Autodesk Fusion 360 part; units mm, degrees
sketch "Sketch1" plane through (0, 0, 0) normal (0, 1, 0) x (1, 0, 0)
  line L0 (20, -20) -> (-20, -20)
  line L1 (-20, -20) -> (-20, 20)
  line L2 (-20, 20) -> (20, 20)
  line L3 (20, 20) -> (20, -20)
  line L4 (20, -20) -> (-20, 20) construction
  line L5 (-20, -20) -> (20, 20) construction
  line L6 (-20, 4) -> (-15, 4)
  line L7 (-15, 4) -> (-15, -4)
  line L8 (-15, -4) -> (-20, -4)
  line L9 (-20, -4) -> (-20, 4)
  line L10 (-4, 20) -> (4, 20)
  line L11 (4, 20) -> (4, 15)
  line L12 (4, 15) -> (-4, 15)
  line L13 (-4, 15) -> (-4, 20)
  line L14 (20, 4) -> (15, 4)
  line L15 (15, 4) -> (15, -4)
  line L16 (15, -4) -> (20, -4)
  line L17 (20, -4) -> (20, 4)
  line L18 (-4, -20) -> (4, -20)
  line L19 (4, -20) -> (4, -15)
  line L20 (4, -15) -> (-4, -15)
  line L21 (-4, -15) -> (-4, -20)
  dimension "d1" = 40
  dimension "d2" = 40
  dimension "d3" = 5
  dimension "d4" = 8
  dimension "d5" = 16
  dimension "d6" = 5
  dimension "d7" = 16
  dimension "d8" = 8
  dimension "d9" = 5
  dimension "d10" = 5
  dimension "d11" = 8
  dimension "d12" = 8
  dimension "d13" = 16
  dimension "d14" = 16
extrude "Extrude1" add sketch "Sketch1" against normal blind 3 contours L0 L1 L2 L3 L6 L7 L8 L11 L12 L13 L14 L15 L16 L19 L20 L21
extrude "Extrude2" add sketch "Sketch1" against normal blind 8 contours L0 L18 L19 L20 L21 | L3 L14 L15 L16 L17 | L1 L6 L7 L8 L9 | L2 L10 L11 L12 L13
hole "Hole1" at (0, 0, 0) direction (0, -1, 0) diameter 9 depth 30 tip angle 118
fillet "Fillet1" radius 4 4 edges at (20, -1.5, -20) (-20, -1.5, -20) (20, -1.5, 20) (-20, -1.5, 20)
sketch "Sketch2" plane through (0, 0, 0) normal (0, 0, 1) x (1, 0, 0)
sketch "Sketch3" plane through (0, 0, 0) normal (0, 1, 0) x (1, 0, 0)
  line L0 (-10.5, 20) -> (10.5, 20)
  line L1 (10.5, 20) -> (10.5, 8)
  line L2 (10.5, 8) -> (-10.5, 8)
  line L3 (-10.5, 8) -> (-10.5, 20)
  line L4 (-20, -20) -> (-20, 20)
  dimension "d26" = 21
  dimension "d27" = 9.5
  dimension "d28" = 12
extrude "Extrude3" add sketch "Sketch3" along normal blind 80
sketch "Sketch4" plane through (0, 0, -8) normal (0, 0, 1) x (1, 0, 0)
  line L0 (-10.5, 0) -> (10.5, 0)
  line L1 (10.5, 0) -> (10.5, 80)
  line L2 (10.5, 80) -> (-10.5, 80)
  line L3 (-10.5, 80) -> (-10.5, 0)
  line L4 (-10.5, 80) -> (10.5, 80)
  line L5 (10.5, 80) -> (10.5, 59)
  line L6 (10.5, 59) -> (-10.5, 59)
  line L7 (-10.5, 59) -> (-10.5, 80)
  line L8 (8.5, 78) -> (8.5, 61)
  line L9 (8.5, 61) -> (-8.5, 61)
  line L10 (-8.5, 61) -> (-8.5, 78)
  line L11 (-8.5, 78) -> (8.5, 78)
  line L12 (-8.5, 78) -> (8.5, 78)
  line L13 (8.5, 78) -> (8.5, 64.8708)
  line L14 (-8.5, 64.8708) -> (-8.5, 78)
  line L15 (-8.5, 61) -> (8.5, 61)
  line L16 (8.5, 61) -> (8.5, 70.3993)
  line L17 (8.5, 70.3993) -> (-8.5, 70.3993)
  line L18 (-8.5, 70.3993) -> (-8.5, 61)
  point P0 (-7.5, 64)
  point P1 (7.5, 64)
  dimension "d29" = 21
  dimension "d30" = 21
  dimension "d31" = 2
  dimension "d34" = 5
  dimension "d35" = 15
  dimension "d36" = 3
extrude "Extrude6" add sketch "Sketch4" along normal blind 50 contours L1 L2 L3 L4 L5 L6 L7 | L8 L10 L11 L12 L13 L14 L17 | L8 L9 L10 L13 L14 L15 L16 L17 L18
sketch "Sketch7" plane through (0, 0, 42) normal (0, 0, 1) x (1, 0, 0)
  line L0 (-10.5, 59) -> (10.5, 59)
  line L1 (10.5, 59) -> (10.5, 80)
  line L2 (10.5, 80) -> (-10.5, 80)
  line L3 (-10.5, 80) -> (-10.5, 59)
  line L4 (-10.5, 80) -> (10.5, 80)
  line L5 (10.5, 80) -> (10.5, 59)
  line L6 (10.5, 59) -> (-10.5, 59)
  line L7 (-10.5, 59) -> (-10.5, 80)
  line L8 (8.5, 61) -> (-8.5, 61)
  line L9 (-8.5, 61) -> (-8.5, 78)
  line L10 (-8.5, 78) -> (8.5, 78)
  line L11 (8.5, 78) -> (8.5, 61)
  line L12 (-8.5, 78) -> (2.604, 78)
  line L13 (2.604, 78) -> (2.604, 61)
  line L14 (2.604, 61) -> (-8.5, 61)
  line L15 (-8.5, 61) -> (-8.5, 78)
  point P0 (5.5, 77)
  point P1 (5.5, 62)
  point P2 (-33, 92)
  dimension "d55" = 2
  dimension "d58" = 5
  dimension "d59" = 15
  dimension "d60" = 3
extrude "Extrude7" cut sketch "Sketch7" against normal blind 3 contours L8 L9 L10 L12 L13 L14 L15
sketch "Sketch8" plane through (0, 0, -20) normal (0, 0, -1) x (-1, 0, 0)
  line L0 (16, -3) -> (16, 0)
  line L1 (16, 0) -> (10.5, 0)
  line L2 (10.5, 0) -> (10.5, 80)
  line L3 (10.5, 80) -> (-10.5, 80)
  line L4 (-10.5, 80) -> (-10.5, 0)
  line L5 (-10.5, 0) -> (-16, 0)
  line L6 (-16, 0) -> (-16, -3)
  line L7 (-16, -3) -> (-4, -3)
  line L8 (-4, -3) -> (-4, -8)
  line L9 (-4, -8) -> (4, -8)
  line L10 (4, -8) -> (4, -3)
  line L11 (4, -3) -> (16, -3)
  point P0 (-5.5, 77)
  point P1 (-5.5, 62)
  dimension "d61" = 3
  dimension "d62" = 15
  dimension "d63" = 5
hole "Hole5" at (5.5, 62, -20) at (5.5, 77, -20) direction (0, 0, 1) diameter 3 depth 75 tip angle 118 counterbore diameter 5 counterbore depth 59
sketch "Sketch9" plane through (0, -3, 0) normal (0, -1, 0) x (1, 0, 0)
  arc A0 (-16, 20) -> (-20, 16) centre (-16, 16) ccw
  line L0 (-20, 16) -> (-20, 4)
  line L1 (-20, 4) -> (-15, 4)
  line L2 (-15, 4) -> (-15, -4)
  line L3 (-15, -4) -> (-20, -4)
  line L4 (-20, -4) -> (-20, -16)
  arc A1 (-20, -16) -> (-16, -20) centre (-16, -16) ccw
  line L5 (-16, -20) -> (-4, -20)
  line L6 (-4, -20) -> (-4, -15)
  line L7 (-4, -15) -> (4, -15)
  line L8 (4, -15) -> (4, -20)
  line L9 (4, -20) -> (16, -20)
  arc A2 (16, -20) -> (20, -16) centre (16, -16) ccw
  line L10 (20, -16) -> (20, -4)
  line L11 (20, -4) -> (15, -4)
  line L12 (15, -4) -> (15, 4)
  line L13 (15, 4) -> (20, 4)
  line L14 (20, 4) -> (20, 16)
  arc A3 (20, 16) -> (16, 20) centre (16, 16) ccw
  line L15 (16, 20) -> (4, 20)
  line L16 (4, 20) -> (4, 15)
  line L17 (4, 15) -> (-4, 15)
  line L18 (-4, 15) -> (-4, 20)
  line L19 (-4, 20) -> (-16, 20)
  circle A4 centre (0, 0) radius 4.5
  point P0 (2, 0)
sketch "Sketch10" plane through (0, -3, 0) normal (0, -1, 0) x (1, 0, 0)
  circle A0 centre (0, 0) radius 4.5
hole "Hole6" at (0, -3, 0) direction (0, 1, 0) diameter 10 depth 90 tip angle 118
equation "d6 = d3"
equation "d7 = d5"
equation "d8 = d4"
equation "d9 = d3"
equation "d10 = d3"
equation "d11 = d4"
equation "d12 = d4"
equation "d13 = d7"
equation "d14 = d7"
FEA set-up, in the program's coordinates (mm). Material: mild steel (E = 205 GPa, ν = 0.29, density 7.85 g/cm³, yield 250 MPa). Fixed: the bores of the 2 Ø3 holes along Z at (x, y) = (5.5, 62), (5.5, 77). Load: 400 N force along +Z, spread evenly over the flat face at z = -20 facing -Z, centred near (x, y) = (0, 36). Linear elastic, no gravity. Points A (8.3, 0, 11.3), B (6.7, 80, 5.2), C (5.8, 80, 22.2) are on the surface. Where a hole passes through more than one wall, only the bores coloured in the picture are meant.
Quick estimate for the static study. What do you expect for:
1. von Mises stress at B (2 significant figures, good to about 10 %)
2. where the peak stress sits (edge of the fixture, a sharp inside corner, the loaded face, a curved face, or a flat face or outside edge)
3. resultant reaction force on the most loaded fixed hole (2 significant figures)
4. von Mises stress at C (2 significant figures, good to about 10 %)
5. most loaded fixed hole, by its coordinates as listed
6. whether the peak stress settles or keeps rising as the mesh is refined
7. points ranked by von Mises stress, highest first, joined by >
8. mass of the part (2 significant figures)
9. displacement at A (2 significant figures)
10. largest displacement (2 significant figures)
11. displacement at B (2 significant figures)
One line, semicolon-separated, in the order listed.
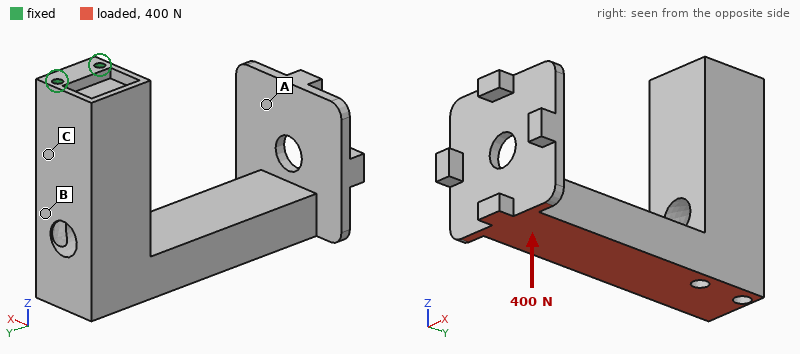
17 MPa; edge of the fixture; 1.0 kN; 12 MPa; (5.5, 62); keeps rising; B > C > A; 340 g; 59 µm; 74 µm; 13 µm
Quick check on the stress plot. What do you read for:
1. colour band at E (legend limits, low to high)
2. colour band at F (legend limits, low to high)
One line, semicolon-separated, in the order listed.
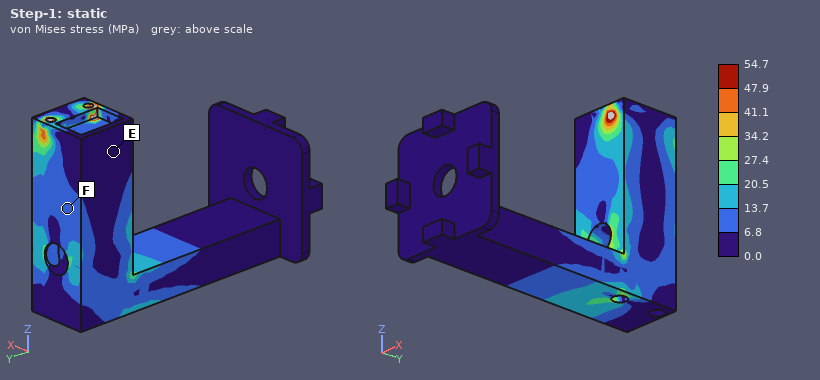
0.0 to 6.8 MPa; 6.8 to 13.7 MPa
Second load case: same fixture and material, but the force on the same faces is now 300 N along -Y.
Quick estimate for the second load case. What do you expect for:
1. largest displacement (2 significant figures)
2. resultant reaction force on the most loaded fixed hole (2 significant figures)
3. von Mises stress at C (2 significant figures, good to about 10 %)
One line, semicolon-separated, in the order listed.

45 µm; 1.2 kN; 12 MPa
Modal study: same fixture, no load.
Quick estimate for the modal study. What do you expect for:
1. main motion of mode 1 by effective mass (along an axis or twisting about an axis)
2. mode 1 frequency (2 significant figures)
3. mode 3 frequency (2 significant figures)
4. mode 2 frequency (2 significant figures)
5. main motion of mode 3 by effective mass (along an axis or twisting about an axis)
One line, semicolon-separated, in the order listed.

along X; 510 Hz; 1400 Hz; 870 Hz; twisting about Z
